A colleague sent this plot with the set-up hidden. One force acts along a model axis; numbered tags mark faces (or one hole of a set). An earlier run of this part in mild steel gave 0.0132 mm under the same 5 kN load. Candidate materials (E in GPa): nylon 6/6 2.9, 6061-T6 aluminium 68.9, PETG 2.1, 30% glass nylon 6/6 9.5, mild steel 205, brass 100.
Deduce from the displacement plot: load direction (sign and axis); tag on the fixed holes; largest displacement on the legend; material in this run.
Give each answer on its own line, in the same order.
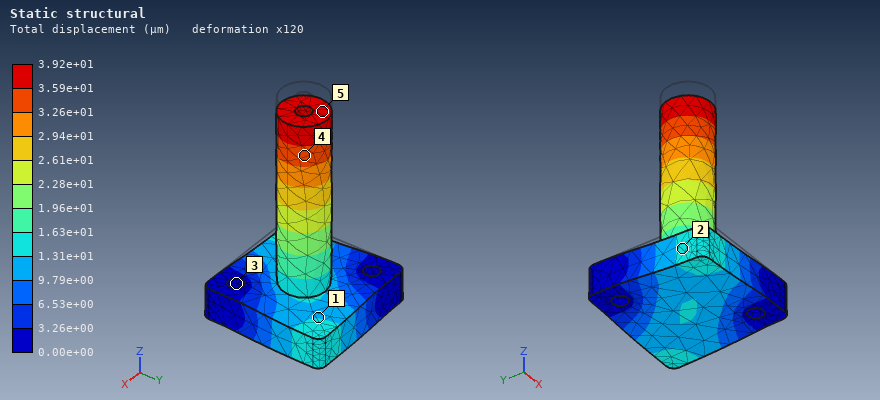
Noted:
-Z
3
3.92e+01 µm
6061-T6 aluminium
